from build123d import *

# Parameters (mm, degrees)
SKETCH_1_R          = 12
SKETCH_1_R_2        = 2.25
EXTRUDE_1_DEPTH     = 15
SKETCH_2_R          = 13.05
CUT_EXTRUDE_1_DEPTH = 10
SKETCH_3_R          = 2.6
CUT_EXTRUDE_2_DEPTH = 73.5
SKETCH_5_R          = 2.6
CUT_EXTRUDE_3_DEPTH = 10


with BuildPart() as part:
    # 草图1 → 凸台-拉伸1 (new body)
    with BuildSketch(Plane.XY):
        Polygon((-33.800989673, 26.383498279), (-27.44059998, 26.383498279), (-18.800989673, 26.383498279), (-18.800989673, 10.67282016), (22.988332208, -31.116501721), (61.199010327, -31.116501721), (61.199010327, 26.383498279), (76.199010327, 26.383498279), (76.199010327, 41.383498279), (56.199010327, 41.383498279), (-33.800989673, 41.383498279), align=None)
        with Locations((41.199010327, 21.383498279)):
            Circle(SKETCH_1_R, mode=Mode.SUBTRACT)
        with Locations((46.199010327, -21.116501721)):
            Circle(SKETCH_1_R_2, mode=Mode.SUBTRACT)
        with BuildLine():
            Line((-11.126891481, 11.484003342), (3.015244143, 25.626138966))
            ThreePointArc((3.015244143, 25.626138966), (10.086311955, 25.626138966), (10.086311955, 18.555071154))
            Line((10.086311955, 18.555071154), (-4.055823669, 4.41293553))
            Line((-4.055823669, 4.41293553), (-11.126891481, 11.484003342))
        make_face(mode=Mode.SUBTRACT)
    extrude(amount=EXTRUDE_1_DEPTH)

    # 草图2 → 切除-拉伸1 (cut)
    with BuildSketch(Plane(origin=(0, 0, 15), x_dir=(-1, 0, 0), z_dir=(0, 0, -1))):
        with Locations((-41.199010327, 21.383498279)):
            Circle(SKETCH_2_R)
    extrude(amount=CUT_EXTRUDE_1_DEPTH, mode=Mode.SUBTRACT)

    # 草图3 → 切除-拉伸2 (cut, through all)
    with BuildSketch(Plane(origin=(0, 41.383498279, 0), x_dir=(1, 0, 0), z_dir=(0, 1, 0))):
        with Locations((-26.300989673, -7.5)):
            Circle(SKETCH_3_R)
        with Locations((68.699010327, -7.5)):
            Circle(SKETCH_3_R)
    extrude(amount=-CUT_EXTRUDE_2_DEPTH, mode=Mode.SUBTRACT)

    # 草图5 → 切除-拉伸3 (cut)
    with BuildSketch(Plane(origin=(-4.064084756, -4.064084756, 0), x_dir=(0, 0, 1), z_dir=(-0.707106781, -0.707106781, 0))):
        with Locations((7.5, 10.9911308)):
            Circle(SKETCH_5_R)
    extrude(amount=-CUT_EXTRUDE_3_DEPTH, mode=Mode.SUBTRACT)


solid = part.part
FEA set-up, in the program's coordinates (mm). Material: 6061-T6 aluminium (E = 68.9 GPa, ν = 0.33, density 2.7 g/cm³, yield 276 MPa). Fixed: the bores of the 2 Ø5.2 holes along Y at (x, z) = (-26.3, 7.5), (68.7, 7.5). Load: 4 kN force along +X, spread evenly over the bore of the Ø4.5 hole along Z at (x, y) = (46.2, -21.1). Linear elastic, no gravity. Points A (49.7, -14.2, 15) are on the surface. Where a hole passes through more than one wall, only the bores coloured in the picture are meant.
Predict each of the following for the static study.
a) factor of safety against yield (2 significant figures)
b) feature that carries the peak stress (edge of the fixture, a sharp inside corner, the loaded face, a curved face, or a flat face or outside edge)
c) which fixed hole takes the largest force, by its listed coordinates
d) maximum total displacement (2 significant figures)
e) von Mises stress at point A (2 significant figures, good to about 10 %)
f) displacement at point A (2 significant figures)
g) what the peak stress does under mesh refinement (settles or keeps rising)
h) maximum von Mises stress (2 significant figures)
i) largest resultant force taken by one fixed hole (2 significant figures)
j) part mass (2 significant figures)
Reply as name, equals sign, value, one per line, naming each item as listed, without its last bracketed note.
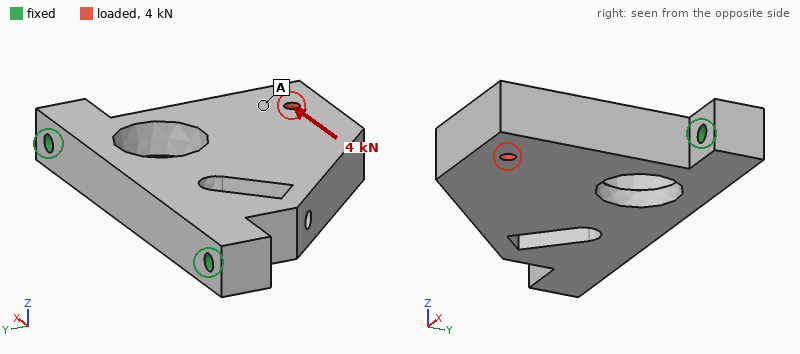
factor of safety against yield = 2.7
feature that carries the peak stress = a curved face
which fixed hole takes the largest force, by its listed coordinates = (-26.3, 7.5)
maximum total displacement = 46 µm
von Mises stress at point A = 11 MPa
displacement at point A = 35 µm
what the peak stress does under mesh refinement = settles
maximum von Mises stress = 100 MPa
largest resultant force taken by one fixed hole = 3.6 kN
part mass = 180 g
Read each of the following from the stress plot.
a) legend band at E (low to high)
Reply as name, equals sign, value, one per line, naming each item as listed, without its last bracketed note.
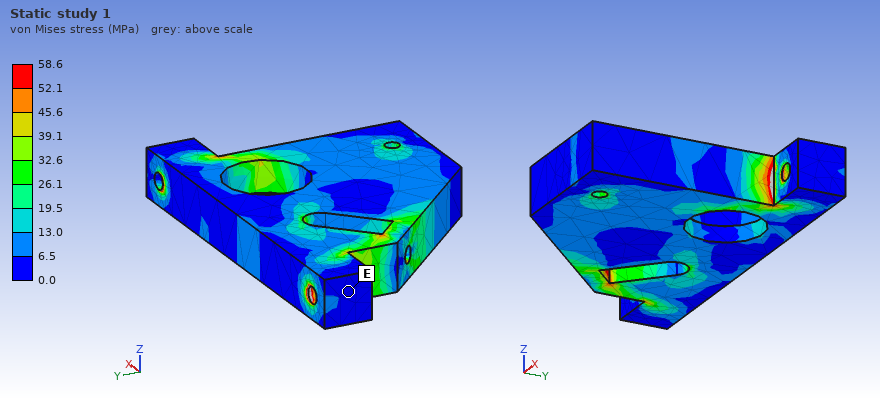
legend band at E = 0.0 to 6.5 MPa
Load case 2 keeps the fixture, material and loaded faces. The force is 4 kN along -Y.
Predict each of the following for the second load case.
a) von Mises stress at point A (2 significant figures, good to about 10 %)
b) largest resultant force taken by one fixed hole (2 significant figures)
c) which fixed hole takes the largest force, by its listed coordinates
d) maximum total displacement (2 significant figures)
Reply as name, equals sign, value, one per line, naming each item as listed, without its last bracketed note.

von Mises stress at point A = 15 MPa
largest resultant force taken by one fixed hole = 3.2 kN
which fixed hole takes the largest force, by its listed coordinates = (68.7, 7.5)
maximum total displacement = 23 µm
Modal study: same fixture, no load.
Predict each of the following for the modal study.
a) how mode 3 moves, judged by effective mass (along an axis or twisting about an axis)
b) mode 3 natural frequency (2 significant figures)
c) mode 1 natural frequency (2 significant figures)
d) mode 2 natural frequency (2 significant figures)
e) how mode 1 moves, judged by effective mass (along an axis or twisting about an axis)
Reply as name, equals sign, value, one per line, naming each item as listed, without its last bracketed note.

how mode 3 moves, judged by effective mass = along X
mode 3 natural frequency = 6100 Hz
mode 1 natural frequency = 1500 Hz
mode 2 natural frequency = 5200 Hz
how mode 1 moves, judged by effective mass = along Z
